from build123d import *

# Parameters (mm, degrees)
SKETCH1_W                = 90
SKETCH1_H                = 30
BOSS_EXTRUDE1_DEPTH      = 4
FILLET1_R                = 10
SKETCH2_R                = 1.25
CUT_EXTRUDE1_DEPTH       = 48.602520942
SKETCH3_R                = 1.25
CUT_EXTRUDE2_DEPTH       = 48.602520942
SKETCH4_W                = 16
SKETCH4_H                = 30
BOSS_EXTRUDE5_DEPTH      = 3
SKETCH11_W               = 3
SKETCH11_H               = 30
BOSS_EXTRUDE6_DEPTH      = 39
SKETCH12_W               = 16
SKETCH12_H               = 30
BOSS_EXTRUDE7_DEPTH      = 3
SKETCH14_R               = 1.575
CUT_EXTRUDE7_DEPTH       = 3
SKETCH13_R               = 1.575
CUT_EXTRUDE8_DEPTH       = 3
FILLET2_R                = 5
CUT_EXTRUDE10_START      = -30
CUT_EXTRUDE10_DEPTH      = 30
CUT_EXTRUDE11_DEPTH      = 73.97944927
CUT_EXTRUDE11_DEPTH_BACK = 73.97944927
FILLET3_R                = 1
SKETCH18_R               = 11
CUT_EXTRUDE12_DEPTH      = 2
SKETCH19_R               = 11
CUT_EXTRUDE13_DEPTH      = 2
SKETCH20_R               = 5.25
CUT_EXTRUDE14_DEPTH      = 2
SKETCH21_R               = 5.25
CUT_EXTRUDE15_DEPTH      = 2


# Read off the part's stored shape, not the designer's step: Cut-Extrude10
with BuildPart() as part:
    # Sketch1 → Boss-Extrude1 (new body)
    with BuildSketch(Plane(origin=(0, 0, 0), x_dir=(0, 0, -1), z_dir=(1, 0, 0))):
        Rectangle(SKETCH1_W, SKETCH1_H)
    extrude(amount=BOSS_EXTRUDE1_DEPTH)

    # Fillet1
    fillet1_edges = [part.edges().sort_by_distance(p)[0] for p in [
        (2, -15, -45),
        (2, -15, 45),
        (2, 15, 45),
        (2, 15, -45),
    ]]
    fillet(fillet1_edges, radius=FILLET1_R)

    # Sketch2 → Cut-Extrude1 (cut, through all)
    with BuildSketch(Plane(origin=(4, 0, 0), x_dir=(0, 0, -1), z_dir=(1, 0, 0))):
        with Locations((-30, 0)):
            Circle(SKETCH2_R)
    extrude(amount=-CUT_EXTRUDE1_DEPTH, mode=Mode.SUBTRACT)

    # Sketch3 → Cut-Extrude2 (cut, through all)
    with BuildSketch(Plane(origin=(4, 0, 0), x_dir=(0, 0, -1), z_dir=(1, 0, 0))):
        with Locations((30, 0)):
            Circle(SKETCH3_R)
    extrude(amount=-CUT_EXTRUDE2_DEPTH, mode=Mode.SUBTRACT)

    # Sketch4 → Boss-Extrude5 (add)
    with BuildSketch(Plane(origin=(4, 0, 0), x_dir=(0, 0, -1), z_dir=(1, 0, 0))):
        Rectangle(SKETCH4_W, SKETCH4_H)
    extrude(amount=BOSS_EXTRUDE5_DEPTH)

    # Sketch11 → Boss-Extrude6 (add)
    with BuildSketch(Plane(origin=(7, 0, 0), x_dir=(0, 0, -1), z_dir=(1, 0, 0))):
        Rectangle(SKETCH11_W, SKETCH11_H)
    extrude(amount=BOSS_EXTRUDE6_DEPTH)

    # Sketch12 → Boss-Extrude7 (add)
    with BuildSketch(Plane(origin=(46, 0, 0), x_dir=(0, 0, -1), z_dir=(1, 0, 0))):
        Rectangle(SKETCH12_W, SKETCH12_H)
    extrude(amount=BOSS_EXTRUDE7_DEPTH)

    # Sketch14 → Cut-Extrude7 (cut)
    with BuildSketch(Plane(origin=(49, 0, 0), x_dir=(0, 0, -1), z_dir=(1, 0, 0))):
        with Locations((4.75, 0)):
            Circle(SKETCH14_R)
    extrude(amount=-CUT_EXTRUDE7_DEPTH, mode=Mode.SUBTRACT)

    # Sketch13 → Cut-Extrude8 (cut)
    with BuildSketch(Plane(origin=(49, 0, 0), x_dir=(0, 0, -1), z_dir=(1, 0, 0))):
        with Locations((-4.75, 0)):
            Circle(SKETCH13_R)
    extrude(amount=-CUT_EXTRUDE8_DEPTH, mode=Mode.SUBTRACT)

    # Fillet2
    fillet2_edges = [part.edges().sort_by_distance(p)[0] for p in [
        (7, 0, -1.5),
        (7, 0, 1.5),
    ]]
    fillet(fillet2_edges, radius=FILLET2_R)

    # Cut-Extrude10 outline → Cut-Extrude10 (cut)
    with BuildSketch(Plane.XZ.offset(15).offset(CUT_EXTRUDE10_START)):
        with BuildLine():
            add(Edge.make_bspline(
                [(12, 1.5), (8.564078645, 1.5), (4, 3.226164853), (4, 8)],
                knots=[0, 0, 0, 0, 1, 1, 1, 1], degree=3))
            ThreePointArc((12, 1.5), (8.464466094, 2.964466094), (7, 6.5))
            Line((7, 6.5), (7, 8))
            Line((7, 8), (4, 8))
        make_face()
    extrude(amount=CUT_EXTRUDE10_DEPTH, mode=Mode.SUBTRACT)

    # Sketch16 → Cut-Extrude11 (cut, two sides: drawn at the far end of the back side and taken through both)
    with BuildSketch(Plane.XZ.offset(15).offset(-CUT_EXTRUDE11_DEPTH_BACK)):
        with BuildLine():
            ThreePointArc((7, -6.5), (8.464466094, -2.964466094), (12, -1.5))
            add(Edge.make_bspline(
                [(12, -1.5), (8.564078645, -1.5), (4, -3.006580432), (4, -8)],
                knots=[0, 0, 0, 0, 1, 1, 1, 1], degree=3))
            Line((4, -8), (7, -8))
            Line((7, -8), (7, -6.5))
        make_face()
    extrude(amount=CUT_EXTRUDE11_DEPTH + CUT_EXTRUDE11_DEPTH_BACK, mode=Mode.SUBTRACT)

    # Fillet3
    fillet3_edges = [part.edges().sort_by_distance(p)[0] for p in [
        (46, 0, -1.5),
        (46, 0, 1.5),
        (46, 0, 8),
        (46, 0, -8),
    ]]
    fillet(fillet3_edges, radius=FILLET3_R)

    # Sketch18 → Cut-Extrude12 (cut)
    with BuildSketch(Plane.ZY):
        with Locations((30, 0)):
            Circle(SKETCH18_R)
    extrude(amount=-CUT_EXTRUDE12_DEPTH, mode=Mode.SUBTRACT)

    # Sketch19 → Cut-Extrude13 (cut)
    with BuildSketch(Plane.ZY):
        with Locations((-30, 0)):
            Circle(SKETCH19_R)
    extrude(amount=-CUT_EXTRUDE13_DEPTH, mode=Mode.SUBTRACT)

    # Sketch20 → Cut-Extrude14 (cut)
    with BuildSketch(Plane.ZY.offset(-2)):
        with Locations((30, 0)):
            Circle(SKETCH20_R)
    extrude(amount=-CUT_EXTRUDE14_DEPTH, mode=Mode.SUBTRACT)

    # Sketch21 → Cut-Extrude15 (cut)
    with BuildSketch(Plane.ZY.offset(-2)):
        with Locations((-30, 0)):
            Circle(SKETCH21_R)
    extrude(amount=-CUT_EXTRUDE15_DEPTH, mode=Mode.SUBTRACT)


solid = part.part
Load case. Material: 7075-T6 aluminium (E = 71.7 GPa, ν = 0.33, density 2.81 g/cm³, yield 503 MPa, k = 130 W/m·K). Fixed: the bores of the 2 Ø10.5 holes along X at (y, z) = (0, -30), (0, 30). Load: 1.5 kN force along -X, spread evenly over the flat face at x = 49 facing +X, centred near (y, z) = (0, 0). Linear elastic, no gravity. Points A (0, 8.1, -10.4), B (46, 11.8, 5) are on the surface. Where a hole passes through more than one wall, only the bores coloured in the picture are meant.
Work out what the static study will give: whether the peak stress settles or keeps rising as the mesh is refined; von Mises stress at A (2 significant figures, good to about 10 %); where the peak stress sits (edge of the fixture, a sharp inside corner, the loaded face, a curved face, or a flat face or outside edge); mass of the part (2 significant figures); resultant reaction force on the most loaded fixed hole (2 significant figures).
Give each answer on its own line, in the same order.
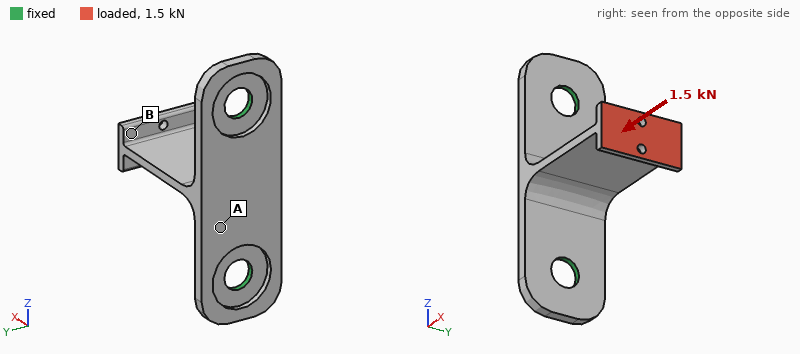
keeps rising
76 MPa
edge of the fixture
40 g
1.3 kN
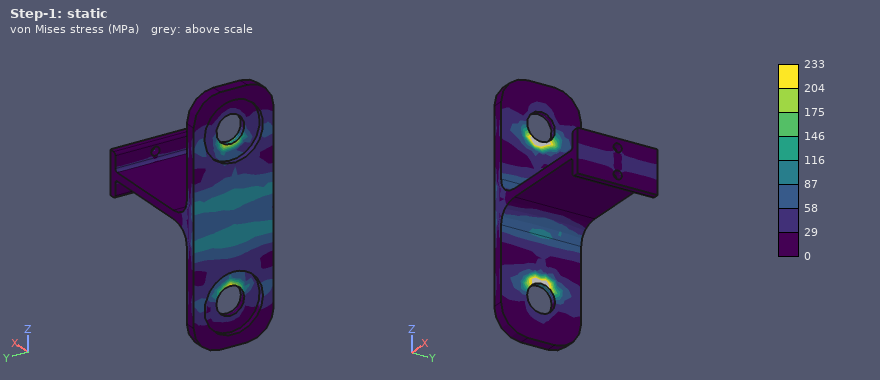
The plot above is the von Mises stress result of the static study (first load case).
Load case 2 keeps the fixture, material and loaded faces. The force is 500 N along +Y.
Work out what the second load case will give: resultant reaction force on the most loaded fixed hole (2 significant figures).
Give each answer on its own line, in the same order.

250 N
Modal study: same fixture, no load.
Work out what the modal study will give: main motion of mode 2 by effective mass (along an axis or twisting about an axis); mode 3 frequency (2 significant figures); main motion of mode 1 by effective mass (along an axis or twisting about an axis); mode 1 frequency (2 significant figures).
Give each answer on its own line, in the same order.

along Y
3100 Hz
along Z
980 Hz
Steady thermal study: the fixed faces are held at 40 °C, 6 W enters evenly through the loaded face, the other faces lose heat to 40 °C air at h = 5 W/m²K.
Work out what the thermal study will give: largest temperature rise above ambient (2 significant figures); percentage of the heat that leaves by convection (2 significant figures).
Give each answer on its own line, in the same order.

27 K
6.1 %
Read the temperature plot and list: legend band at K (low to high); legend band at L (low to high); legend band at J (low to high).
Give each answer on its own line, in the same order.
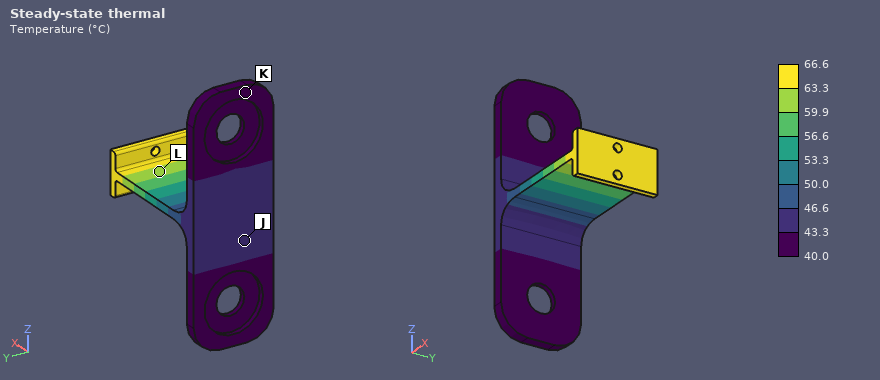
40.0 to 43.3 °C
59.9 to 63.3 °C
43.3 to 46.6 °C
